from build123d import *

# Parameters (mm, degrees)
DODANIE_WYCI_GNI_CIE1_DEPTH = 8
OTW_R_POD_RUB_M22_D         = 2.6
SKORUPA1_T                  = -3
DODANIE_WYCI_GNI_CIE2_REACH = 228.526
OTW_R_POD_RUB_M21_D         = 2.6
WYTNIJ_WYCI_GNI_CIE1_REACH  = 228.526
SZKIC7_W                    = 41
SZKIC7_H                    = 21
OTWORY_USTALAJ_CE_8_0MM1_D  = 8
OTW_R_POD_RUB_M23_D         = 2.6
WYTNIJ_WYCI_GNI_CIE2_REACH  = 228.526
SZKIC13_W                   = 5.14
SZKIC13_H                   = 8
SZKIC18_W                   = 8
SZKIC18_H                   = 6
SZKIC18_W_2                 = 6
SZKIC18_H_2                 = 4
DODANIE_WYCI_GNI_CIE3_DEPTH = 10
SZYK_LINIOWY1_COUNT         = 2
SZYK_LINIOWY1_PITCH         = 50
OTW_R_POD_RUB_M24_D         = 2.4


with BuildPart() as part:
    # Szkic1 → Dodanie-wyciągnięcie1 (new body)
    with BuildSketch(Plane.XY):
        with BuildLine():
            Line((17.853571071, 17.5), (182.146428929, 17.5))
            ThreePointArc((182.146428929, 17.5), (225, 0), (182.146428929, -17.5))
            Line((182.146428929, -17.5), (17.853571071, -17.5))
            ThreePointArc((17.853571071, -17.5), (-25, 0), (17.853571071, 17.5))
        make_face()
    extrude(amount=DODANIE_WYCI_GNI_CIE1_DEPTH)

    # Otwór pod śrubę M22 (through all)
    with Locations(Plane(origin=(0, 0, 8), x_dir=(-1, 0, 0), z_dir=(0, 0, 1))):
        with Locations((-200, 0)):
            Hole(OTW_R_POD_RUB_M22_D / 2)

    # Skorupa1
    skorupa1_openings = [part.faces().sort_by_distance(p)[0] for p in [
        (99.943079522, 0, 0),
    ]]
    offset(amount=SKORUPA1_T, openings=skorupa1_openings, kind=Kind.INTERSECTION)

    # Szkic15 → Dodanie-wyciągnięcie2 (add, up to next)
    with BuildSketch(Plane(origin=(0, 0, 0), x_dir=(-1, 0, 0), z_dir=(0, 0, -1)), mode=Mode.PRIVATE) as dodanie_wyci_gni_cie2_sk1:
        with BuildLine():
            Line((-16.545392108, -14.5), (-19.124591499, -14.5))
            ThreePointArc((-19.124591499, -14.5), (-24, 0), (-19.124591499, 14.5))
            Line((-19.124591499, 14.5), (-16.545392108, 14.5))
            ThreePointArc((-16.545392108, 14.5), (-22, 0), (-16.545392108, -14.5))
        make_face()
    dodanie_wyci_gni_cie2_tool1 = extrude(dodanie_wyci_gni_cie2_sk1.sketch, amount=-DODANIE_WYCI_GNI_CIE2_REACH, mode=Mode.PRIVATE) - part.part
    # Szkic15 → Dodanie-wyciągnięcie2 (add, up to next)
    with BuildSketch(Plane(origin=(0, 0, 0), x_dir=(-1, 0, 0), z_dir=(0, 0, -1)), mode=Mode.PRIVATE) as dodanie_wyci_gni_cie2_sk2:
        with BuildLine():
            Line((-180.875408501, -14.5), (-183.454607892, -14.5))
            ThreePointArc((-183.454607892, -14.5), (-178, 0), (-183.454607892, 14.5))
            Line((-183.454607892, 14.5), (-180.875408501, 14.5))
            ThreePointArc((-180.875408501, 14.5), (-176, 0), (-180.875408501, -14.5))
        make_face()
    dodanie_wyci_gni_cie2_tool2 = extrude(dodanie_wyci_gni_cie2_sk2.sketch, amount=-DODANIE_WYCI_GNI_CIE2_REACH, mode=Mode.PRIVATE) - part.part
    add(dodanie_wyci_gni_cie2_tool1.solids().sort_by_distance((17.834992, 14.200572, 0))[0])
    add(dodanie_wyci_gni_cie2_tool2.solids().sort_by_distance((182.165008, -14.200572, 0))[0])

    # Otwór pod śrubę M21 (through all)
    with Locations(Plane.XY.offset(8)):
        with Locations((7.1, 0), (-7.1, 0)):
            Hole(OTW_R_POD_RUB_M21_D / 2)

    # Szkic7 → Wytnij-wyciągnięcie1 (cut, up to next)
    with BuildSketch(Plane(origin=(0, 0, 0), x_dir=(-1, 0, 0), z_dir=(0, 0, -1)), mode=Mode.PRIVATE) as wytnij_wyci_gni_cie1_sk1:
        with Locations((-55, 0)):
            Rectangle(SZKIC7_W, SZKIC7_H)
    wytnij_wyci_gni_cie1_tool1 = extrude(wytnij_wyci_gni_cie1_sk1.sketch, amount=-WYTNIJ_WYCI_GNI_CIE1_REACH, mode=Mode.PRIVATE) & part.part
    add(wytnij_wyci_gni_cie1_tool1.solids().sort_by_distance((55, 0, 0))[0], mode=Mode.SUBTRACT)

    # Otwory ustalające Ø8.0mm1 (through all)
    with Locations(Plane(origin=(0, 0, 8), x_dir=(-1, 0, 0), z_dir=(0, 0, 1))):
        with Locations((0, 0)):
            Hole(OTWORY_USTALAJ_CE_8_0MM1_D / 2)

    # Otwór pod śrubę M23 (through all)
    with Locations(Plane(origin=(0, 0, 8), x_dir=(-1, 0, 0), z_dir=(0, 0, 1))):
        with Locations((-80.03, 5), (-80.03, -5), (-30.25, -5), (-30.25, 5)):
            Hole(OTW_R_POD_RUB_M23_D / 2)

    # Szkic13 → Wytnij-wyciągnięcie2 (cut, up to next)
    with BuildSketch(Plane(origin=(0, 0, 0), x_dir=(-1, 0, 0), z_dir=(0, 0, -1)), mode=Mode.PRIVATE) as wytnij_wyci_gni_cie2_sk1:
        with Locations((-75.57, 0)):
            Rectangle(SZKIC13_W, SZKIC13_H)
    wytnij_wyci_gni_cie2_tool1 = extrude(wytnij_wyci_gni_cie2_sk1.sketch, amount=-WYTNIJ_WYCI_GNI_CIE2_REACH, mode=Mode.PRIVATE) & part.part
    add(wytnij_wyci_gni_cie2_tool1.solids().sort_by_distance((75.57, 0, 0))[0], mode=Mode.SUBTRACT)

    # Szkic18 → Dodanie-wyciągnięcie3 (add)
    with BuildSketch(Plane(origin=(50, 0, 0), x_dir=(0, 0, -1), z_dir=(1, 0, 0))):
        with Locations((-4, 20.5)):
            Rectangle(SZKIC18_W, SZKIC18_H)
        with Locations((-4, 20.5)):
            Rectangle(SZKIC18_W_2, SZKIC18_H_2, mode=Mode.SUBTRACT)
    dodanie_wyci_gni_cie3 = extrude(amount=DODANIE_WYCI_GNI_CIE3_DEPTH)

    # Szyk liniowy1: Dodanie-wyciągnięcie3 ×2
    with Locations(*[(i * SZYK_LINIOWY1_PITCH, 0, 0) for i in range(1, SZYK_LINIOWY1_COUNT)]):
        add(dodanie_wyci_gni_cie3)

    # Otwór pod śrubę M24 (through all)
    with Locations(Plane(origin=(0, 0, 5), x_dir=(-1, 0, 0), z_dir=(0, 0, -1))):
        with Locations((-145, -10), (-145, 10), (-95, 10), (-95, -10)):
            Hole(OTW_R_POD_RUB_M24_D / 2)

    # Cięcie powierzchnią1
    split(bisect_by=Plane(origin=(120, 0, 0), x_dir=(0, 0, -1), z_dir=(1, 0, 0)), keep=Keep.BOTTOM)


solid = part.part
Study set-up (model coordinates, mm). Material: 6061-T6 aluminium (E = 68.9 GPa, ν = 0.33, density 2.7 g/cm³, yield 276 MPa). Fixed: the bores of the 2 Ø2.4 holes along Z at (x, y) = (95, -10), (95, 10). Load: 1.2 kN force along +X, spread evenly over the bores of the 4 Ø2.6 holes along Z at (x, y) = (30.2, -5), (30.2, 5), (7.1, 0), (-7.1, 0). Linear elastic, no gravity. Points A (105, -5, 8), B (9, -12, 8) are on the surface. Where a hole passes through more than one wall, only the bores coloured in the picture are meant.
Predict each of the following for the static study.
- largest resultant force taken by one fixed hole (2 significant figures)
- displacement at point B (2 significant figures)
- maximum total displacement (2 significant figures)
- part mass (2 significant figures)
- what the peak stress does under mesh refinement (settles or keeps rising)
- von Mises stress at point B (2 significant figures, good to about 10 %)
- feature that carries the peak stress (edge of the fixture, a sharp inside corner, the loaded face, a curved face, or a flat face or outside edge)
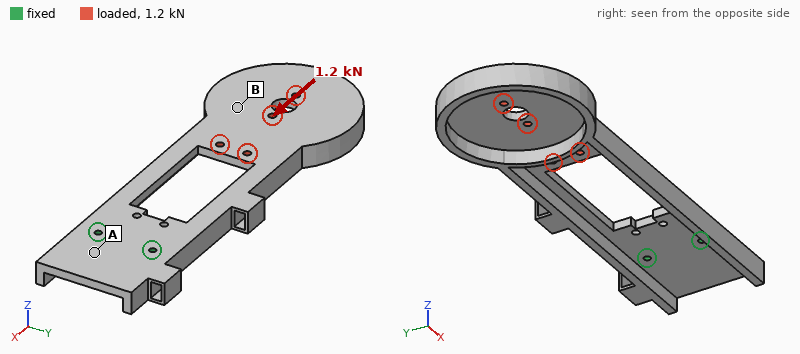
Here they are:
600 N
0.23 mm
0.39 mm
51 g
keeps rising
6.1 MPa
edge of the fixture
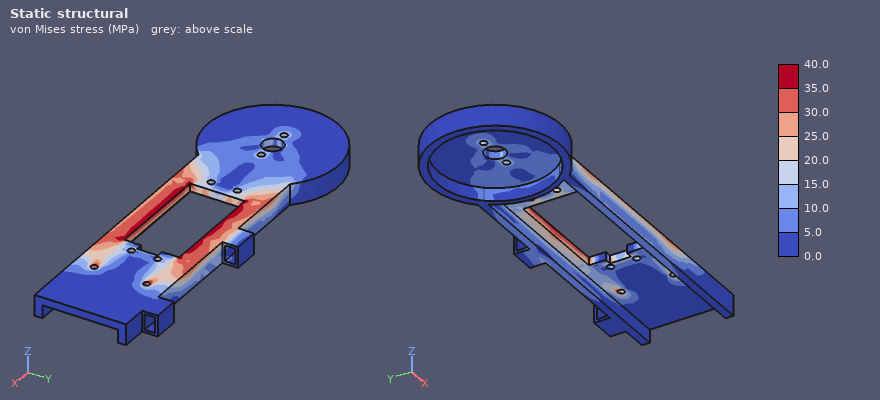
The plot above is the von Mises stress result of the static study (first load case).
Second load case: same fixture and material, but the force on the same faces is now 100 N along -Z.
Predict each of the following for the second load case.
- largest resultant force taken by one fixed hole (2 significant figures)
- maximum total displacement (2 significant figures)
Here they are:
60 N
1.6 mm
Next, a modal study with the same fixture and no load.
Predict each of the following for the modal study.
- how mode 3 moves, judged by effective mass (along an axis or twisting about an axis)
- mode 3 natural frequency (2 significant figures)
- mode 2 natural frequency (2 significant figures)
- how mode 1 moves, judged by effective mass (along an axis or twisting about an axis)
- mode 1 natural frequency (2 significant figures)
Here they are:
along Y
980 Hz
750 Hz
along Z
260 Hz
